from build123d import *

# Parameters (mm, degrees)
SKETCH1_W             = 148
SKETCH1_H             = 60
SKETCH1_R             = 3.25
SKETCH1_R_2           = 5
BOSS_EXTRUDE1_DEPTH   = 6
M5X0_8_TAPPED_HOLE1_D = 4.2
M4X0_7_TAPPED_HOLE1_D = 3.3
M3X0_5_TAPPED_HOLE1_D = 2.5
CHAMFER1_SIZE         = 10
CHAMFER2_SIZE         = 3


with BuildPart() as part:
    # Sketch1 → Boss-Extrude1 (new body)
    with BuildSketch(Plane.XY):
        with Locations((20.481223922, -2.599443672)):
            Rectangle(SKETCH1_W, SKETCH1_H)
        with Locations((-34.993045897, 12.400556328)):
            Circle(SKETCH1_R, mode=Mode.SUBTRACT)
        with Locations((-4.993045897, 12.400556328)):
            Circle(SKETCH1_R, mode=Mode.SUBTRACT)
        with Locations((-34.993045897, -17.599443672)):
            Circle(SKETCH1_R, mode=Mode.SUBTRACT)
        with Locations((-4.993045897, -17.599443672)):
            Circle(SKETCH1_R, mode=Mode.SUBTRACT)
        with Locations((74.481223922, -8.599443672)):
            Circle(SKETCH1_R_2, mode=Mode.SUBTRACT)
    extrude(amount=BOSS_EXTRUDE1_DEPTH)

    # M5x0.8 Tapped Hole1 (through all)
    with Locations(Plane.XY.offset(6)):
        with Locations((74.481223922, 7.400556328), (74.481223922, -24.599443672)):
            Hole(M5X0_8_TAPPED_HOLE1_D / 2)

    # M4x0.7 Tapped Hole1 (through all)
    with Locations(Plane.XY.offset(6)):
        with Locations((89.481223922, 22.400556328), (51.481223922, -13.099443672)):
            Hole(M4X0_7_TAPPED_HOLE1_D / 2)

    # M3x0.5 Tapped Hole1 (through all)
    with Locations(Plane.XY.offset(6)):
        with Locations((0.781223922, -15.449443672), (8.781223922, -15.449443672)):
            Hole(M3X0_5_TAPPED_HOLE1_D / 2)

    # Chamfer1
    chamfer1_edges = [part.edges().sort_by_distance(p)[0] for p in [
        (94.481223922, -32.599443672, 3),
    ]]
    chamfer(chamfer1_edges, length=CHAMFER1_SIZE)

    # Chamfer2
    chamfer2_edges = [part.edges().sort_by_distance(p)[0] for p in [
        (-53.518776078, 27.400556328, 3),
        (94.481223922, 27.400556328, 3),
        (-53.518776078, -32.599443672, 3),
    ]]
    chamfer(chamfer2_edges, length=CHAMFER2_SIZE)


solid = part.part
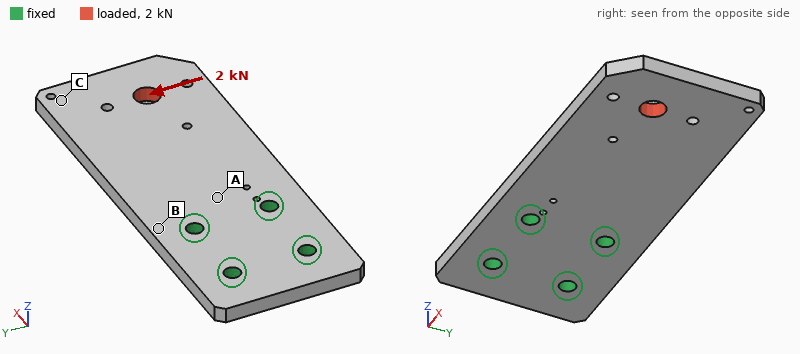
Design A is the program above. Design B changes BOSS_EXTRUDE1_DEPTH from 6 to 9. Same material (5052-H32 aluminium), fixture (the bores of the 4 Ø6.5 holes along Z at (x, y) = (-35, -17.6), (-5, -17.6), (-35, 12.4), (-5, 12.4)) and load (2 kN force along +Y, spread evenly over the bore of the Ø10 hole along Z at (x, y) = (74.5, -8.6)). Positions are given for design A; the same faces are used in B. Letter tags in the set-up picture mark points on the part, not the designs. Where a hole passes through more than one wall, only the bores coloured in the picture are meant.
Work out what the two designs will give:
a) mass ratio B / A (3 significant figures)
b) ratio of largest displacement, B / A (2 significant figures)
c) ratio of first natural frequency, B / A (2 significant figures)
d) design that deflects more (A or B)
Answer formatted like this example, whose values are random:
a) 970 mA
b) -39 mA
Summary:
a) 1.50
b) 0.67
c) 1.5
d) A
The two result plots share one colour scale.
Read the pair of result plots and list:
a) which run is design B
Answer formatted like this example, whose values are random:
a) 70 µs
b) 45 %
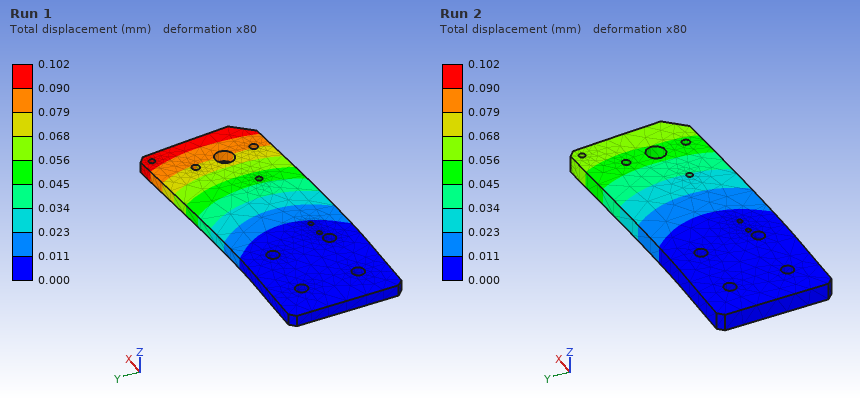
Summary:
a) Run 2
